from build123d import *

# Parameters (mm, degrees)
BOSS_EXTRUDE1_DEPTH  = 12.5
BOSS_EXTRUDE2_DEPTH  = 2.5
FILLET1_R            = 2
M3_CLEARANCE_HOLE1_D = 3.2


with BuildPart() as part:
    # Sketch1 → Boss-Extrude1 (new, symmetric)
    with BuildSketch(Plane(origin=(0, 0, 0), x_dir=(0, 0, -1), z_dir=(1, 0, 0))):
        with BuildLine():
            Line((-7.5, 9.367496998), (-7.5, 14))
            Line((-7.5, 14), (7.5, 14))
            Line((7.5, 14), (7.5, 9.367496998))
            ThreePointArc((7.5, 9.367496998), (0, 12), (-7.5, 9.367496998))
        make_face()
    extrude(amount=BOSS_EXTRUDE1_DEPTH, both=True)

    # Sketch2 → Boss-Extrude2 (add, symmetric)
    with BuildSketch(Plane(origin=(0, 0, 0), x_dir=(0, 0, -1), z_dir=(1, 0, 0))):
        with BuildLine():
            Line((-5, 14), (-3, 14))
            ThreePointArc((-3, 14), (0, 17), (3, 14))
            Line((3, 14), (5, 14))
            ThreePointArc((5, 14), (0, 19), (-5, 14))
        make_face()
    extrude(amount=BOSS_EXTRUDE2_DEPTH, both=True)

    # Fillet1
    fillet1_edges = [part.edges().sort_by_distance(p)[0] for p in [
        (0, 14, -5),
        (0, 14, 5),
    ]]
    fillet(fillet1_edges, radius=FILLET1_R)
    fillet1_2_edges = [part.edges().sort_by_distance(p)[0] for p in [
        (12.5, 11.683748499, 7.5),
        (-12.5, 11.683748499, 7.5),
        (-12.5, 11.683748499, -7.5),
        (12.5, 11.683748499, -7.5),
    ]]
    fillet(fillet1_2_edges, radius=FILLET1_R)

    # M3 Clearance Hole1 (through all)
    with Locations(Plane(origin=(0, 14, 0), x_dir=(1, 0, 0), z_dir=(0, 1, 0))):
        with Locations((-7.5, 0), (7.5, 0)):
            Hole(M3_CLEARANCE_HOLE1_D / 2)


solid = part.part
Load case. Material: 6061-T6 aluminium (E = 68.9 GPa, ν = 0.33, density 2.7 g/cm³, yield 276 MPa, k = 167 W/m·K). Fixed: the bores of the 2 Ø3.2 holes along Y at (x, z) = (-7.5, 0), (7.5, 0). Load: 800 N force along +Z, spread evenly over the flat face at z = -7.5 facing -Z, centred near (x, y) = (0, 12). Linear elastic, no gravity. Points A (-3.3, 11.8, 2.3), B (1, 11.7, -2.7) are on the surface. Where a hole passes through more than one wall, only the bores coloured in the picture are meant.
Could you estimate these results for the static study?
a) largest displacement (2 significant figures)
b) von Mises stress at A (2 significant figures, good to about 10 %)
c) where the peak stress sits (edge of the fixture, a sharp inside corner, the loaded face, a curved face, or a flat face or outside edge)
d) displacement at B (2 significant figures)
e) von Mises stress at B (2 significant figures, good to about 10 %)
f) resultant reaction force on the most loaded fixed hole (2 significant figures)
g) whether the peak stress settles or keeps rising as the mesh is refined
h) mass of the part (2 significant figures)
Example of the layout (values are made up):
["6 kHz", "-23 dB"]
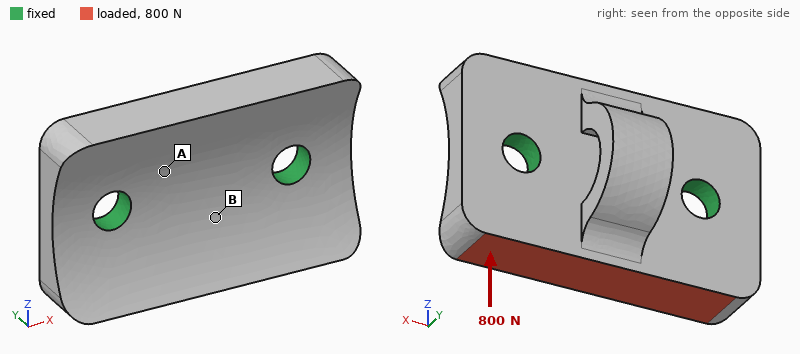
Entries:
["18 µm", "11 MPa", "edge of the fixture", "5.0 µm", "31 MPa", "410 N", "keeps rising", "3.1 g"]
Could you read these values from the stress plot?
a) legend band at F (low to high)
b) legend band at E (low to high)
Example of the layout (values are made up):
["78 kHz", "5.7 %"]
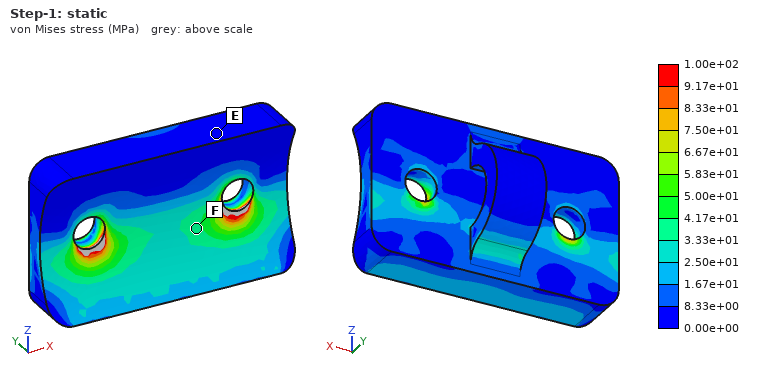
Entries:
["3.33e+01 to 4.17e+01 MPa", "0.00e+00 to 8.33e+00 MPa"]
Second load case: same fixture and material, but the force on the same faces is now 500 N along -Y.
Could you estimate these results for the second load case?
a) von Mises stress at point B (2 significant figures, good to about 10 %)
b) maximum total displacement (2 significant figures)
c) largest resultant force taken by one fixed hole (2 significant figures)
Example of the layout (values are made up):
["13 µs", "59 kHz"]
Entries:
["51 MPa", "45 µm", "250 N"]
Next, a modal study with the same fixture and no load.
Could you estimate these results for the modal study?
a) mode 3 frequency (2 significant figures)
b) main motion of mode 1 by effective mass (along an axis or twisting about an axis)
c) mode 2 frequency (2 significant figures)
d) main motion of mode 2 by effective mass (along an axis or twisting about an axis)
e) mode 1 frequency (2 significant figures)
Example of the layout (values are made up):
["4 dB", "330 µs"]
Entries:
["35 kHz", "twisting about X", "28 kHz", "along Y", "22 kHz"]
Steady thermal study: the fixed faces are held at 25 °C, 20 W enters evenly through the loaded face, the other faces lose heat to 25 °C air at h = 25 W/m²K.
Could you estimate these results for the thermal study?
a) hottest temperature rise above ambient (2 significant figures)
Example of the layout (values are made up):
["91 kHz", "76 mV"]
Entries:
["18 K"]
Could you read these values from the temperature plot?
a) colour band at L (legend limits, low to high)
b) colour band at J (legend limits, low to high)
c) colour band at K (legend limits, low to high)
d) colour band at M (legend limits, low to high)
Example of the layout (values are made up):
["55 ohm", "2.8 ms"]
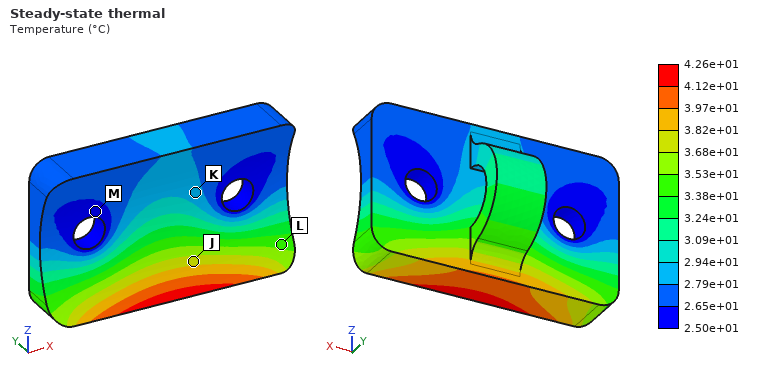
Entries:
["3.38e+01 to 3.53e+01 °C", "3.68e+01 to 3.82e+01 °C", "2.79e+01 to 2.94e+01 °C", "2.50e+01 to 2.65e+01 °C"]
